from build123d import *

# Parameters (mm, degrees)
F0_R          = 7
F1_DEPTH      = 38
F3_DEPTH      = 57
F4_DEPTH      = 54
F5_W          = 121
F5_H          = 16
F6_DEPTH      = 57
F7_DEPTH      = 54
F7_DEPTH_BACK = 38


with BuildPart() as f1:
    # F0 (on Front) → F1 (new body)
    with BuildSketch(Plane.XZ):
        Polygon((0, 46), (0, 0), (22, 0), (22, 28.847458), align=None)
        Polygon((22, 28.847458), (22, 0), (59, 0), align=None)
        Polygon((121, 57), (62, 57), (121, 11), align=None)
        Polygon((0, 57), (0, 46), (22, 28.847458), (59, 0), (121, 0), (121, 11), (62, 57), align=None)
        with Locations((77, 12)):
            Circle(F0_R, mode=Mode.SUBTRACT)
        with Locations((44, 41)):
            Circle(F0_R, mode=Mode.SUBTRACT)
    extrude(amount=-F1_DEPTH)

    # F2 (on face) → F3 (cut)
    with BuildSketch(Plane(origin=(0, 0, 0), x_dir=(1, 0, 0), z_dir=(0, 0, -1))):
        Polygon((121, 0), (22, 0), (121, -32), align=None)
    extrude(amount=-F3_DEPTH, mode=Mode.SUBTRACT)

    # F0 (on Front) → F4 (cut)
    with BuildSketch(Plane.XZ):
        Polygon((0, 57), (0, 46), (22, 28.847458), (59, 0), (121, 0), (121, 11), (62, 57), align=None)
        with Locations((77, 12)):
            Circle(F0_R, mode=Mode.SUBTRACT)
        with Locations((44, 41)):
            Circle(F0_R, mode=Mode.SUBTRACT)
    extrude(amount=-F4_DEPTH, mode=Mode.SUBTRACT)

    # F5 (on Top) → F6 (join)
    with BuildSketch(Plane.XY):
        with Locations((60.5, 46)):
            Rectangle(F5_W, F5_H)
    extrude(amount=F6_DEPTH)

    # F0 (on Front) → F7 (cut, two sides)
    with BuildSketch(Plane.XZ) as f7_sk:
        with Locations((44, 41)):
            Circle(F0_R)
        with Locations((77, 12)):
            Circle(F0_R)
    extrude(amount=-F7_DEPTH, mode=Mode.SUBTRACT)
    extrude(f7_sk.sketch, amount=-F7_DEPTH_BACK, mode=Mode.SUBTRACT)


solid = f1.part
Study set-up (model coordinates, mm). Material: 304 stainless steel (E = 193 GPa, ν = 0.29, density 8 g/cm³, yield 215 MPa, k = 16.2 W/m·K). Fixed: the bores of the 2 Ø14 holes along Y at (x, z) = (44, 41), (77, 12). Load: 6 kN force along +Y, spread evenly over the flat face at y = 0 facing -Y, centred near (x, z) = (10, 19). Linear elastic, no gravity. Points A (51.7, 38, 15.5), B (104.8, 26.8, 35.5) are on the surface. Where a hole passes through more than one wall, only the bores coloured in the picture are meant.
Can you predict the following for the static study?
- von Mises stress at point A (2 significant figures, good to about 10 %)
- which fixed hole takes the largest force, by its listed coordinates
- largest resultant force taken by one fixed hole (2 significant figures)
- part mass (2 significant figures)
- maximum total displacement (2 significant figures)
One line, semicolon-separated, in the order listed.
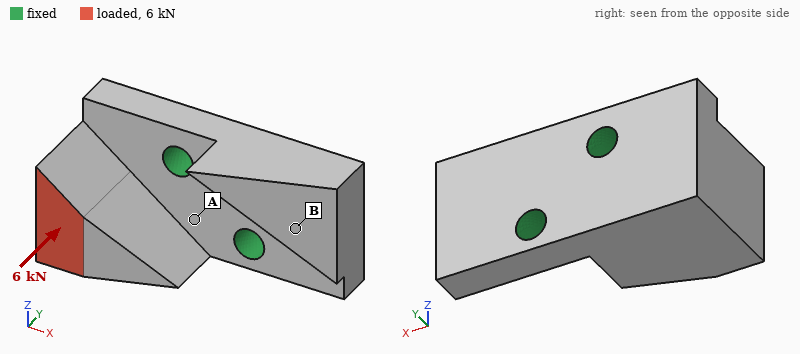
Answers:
44 MPa; (44, 41); 6.4 kN; 1.4 kg; 73 µm
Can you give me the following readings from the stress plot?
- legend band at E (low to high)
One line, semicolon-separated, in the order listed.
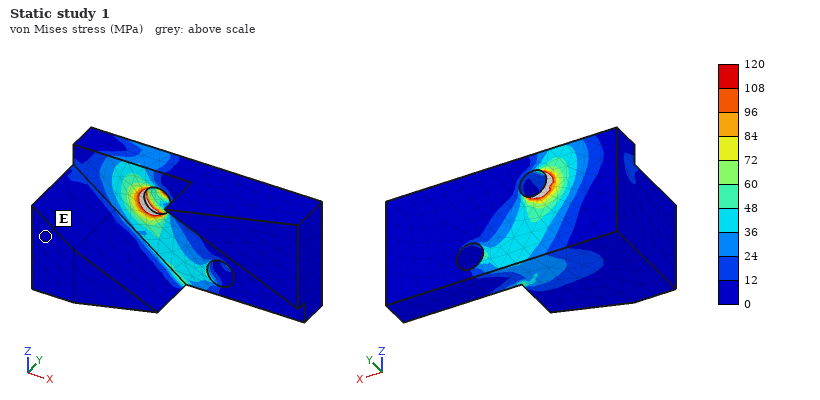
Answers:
0 to 12 MPa
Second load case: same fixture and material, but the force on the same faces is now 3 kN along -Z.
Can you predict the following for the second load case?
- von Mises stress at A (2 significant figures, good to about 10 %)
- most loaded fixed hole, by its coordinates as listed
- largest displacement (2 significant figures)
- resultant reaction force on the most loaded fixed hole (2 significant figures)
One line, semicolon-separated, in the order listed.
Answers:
29 MPa; (44, 41); 53 µm; 4.3 kN
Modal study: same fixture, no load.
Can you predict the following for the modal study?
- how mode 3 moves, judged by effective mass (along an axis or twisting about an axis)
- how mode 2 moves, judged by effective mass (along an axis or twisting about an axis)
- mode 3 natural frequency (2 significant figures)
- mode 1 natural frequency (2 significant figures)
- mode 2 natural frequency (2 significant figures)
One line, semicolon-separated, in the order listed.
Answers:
along Z; along Y; 4500 Hz; 2300 Hz; 3800 Hz
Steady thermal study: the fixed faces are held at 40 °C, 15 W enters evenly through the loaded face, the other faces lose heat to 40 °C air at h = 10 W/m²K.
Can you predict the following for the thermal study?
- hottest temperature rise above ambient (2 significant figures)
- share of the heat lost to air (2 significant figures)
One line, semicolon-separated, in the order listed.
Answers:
56 K; 23 %
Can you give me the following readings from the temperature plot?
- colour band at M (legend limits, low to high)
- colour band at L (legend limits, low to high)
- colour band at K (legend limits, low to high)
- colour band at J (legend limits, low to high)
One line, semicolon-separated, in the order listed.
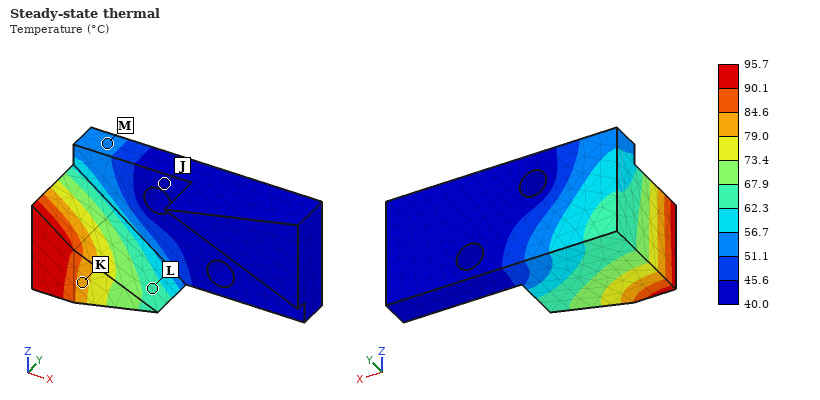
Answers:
51.1 to 56.7 °C; 62.3 to 67.9 °C; 79.0 to 84.6 °C; 40.0 to 45.6 °C
